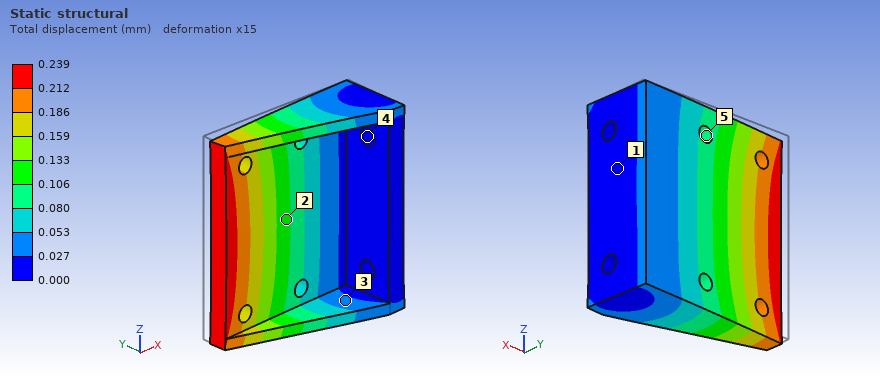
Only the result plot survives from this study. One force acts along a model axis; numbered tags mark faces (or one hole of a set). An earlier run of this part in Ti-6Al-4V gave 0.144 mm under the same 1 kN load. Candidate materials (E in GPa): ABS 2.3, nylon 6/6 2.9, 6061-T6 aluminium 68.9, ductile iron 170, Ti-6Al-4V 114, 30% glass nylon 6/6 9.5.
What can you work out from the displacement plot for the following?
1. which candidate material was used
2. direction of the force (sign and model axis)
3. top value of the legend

6061-T6 aluminium
-Y
0.239 mm
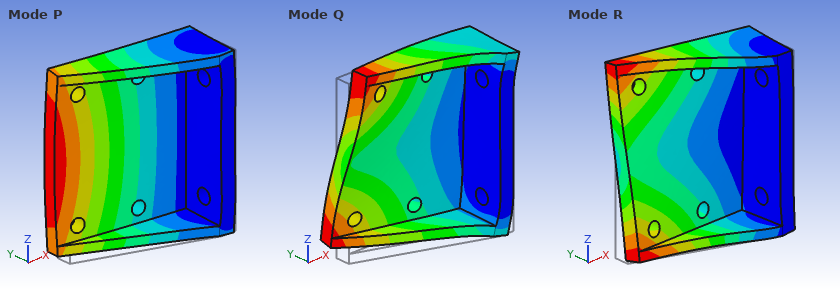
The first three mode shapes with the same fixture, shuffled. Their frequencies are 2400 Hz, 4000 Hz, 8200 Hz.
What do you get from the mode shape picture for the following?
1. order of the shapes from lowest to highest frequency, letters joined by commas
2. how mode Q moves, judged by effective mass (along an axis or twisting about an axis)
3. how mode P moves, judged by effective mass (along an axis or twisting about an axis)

P, R, Q
along Z
along Y
